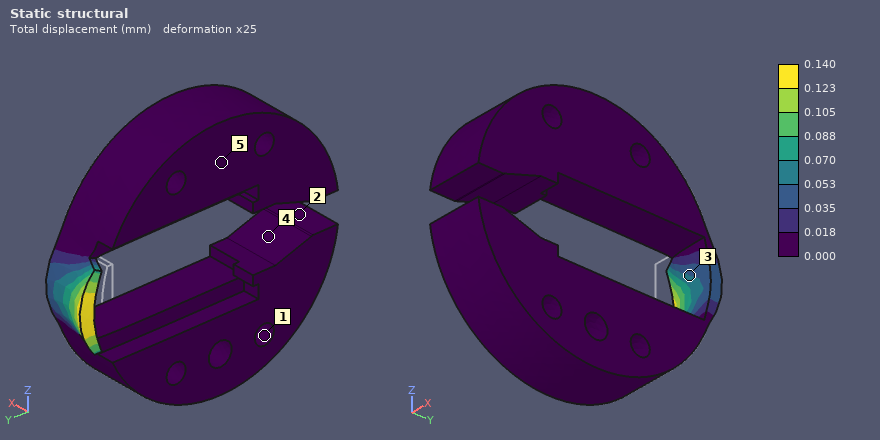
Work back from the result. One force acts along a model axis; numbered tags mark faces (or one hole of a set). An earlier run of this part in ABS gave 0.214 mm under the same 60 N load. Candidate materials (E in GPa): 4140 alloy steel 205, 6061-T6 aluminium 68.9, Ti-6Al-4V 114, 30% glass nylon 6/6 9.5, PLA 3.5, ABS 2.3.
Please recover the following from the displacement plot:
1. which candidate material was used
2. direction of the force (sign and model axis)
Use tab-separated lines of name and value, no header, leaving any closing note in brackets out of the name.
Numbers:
which candidate material was used	PLA
direction of the force	+Y
